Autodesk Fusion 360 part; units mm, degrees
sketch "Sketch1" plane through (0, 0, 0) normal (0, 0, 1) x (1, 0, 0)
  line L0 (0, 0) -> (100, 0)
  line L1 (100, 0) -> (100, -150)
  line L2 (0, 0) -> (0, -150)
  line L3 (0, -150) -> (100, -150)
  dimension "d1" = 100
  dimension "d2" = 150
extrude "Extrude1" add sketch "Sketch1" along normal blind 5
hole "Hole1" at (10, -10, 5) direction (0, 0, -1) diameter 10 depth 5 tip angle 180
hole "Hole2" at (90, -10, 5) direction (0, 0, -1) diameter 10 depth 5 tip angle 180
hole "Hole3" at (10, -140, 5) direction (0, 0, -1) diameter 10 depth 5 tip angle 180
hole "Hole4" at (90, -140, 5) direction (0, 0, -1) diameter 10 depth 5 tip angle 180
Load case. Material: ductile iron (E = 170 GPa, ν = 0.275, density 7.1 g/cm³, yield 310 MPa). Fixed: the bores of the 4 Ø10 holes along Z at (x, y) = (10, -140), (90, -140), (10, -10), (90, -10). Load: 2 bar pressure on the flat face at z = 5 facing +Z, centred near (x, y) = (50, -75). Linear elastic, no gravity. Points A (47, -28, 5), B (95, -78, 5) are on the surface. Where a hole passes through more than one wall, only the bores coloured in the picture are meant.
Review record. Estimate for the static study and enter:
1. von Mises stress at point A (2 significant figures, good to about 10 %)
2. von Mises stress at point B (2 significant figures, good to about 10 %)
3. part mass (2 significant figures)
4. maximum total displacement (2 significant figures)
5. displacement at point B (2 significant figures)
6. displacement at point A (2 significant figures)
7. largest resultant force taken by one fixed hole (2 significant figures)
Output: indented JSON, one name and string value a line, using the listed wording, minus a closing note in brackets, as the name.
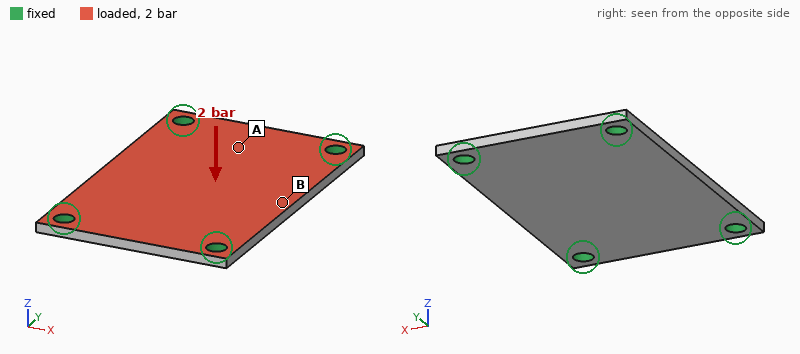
{
  "von Mises stress at point A": "19 MPa",
  "von Mises stress at point B": "38 MPa",
  "part mass": "520 g",
  "maximum total displacement": "0.10 mm",
  "displacement at point B": "0.089 mm",
  "displacement at point A": "0.041 mm",
  "largest resultant force taken by one fixed hole": "730 N"
}
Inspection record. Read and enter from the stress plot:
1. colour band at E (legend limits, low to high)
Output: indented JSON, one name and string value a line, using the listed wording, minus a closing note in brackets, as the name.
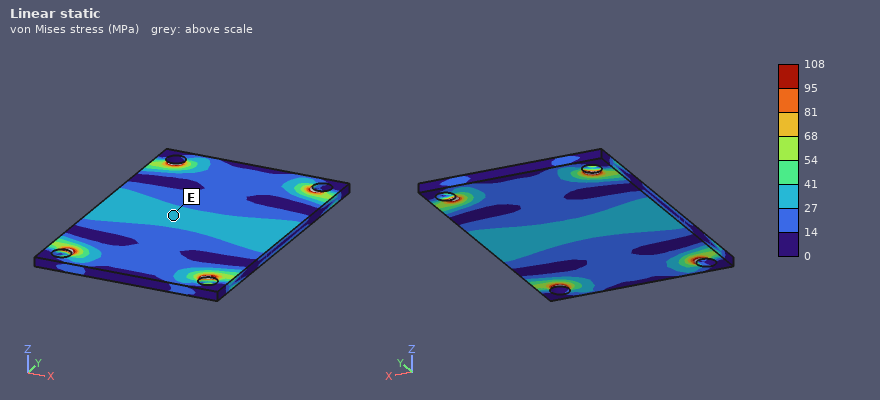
{
  "colour band at E": "27 to 41 MPa"
}
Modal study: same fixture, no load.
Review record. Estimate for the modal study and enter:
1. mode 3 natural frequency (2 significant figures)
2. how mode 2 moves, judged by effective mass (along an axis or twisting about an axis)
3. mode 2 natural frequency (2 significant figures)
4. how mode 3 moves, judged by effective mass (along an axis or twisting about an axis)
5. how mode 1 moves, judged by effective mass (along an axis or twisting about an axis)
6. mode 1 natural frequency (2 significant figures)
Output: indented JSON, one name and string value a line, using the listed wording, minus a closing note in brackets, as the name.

{
  "mode 3 natural frequency": "3500 Hz",
  "how mode 2 moves, judged by effective mass": "twisting about Y",
  "mode 2 natural frequency": "2100 Hz",
  "how mode 3 moves, judged by effective mass": "twisting about X",
  "how mode 1 moves, judged by effective mass": "along Z",
  "mode 1 natural frequency": "1400 Hz"
}
